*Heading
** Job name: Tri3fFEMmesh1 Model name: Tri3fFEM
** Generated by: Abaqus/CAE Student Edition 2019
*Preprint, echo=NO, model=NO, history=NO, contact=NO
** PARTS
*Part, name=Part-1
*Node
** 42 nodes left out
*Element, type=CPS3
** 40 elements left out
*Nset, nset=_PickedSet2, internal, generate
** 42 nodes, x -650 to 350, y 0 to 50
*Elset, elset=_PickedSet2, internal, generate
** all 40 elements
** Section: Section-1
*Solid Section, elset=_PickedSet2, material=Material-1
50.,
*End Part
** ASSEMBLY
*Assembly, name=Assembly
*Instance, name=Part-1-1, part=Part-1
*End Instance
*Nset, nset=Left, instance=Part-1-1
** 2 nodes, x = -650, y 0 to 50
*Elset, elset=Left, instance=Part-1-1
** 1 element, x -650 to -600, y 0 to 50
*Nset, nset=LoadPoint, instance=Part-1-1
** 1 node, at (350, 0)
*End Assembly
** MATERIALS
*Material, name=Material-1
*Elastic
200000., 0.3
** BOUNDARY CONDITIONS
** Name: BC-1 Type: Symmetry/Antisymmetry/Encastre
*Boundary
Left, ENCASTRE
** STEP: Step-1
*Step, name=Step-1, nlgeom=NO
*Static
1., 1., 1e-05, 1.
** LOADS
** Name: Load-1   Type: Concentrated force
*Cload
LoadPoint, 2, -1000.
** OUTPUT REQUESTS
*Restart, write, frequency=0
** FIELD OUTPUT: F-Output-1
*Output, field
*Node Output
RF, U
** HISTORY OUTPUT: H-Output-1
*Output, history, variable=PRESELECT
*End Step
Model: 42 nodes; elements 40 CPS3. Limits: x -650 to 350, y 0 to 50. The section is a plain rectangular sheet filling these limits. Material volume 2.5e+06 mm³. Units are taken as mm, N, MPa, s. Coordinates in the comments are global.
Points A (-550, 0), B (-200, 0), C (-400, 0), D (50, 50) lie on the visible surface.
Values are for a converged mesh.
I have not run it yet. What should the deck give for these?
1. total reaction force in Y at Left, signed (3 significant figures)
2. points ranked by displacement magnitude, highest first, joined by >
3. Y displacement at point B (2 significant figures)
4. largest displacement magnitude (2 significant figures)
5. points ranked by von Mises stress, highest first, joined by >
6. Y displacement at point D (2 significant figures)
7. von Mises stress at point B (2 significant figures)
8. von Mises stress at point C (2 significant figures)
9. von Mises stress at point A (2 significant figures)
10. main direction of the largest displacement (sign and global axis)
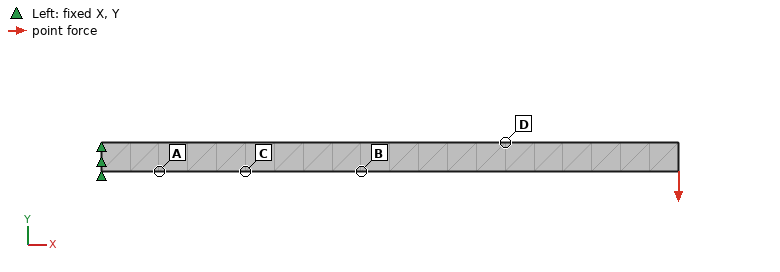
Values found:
1000 N
D > B > C > A
-0.81 mm
3.1 mm
A > C > B > D
-1.8 mm
25 MPa
35 MPa
42 MPa
-Y
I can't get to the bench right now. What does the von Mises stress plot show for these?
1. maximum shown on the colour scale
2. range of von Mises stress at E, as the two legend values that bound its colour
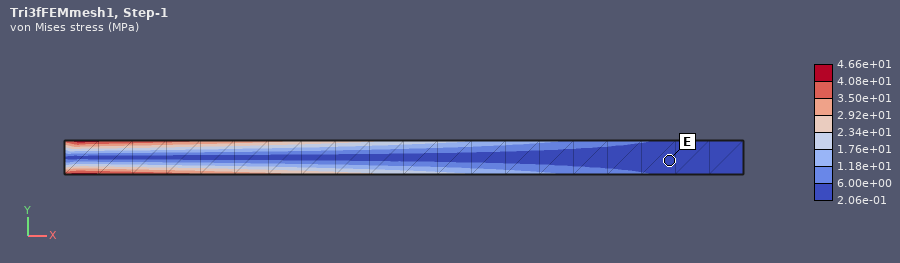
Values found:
4.66e+01 MPa
2.06e-01 to 6.00e+00 MPa
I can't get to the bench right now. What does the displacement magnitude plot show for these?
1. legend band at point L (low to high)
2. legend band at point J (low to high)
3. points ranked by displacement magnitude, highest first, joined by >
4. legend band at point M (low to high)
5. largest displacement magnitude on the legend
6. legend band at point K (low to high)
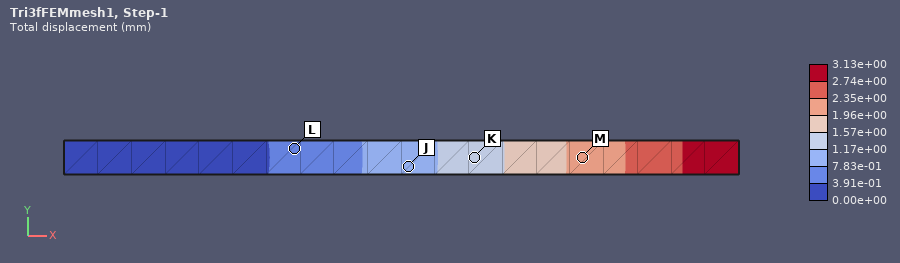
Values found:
3.91e-01 to 7.83e-01 mm
7.83e-01 to 1.17e+00 mm
M > K > J > L
1.96e+00 to 2.35e+00 mm
3.13e+00 mm
1.17e+00 to 1.57e+00 mm
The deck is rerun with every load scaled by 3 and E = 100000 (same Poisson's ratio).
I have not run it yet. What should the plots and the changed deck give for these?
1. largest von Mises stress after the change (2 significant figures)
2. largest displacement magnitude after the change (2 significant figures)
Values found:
140 MPa
19 mm
